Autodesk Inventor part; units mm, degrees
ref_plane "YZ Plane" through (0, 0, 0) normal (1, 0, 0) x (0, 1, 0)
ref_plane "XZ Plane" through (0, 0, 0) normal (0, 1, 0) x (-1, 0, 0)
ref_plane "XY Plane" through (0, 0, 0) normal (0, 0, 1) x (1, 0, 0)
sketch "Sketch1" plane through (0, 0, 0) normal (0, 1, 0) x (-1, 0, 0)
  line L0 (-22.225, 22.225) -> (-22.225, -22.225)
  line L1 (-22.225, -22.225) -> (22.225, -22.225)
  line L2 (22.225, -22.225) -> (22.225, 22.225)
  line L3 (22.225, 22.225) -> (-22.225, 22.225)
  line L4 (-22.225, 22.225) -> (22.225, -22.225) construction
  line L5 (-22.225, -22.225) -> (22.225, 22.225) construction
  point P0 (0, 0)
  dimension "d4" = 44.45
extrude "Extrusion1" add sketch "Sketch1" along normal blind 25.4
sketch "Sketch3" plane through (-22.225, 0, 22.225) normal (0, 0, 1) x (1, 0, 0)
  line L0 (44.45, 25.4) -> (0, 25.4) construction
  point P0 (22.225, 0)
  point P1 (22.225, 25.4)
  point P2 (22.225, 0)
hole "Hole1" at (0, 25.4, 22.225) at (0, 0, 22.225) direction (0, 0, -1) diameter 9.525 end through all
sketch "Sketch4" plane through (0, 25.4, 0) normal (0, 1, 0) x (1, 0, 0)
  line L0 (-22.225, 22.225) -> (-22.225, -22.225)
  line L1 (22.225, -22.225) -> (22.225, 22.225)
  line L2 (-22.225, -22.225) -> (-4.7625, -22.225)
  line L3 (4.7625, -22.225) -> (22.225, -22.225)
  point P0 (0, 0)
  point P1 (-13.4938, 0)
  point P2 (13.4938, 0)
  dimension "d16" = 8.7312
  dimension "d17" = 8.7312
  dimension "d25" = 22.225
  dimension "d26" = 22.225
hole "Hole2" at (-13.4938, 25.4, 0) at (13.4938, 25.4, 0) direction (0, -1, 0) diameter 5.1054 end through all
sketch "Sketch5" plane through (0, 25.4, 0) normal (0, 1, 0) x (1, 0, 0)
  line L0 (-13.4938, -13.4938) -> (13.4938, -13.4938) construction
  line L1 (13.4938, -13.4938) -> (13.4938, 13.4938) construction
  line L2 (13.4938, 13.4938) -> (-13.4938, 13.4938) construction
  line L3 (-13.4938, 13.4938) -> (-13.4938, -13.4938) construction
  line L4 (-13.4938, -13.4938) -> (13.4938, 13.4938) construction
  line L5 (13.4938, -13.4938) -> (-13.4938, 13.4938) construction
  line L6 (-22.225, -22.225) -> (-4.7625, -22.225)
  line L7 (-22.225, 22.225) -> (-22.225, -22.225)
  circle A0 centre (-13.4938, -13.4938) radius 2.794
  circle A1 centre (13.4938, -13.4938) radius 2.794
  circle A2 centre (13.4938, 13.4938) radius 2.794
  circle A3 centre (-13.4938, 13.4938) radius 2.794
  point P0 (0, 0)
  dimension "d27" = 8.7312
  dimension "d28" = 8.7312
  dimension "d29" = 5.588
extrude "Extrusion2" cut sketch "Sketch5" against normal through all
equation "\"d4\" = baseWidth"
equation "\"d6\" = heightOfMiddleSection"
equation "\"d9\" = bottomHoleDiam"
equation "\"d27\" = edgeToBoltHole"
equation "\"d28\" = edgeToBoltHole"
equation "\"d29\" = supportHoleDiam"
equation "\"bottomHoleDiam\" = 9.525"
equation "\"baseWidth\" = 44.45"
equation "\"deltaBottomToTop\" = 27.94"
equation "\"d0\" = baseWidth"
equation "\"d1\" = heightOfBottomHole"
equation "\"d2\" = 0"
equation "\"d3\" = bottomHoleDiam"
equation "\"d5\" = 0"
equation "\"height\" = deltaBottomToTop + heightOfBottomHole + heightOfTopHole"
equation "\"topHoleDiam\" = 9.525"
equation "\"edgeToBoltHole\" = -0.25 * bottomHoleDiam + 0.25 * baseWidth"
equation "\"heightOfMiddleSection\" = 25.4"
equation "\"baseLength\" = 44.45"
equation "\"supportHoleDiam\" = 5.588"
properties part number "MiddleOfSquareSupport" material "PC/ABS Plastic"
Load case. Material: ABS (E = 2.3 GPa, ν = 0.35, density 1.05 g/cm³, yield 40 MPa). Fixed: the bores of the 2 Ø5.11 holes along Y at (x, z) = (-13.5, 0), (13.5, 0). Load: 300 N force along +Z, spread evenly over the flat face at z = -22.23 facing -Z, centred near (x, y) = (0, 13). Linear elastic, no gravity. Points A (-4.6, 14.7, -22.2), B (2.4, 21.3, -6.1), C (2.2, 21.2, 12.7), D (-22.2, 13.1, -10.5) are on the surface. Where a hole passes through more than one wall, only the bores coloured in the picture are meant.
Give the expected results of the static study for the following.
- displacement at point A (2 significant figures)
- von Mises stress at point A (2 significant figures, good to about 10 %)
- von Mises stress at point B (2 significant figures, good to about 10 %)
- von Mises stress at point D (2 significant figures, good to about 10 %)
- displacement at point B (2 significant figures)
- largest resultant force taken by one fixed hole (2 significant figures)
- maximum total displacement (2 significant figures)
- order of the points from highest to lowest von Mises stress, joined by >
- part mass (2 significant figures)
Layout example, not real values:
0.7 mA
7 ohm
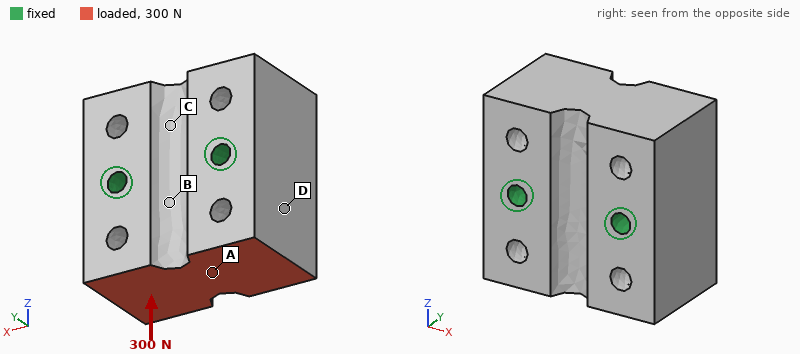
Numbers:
3.3 µm
0.35 MPa
0.19 MPa
0.25 MPa
1.6 µm
150 N
4.2 µm
A > D > B > C
46 g
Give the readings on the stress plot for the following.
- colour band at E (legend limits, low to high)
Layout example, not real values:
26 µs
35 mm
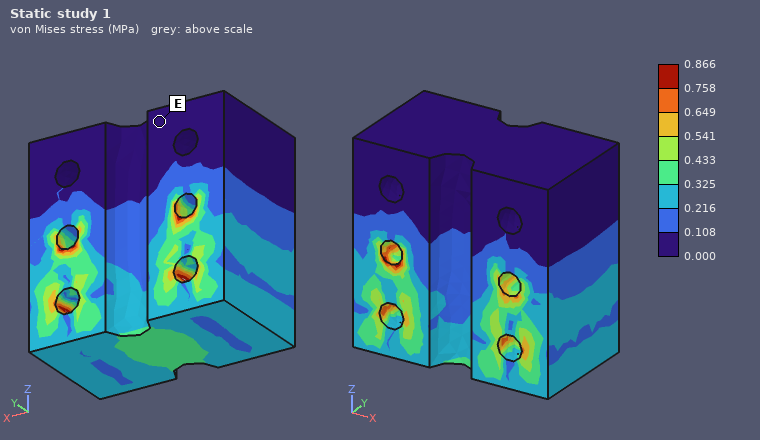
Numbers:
0.000 to 0.108 MPa
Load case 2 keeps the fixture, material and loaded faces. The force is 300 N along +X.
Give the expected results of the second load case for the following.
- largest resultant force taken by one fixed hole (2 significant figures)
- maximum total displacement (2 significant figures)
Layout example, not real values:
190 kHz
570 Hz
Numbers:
260 N
19 µm
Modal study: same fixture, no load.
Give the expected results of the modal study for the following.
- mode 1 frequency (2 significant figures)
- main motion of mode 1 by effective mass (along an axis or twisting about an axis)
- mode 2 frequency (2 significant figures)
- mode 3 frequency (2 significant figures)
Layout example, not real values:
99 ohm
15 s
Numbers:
6300 Hz
twisting about X
7100 Hz
7200 Hz
